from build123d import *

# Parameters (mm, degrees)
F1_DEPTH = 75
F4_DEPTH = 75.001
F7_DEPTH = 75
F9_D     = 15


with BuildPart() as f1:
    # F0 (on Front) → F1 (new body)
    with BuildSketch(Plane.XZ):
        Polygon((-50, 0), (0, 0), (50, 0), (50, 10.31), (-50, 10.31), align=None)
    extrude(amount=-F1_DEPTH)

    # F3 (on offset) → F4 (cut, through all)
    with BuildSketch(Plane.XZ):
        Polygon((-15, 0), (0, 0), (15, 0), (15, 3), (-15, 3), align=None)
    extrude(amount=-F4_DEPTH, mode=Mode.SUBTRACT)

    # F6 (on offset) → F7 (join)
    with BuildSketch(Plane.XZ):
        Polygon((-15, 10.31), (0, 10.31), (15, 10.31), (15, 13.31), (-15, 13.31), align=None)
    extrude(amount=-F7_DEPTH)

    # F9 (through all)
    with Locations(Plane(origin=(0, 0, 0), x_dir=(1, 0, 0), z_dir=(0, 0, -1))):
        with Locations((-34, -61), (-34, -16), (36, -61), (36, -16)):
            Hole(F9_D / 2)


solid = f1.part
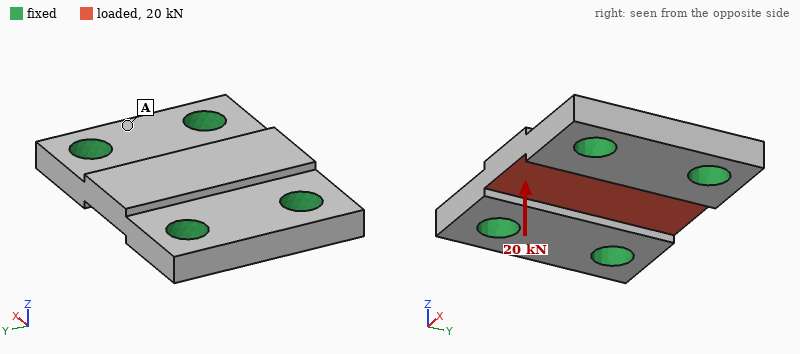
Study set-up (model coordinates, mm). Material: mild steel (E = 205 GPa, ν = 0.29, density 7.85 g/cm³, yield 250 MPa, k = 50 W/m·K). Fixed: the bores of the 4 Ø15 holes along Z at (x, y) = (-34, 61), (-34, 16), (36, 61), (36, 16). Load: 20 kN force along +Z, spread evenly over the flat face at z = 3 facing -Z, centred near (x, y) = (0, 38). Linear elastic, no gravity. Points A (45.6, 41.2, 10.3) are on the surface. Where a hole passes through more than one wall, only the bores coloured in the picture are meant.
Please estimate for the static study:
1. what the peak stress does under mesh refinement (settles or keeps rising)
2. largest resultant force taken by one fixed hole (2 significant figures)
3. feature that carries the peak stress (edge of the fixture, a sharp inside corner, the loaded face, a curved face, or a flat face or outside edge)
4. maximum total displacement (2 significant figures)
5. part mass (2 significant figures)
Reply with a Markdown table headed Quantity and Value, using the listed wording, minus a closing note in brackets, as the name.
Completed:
| Quantity | Value |
|---|---|
| what the peak stress does under mesh refinement | keeps rising |
| largest resultant force taken by one fixed hole | 6.6 kN |
| feature that carries the peak stress | edge of the fixture |
| maximum total displacement | 18 µm |
| part mass | 550 g |
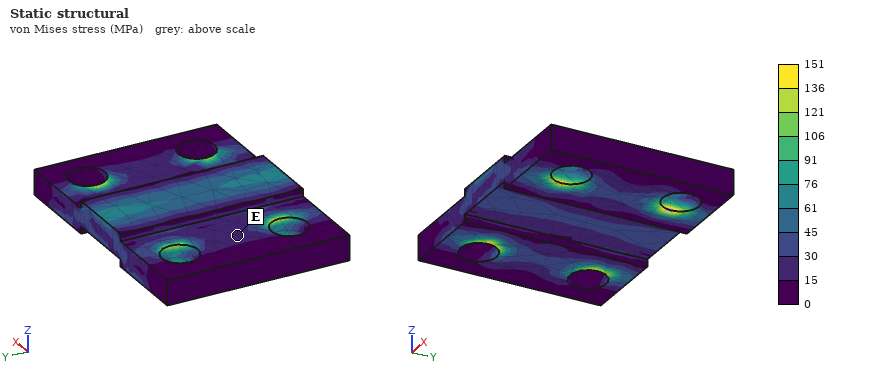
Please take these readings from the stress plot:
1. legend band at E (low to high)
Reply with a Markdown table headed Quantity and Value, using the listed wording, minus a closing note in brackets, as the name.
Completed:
| Quantity | Value |
|---|---|
| legend band at E | 15 to 30 MPa |
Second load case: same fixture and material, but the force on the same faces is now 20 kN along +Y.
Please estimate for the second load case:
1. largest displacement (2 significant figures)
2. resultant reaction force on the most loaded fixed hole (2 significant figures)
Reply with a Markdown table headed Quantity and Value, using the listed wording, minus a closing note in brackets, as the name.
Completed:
| Quantity | Value |
|---|---|
| largest displacement | 7.9 µm |
| resultant reaction force on the most loaded fixed hole | 5.6 kN |
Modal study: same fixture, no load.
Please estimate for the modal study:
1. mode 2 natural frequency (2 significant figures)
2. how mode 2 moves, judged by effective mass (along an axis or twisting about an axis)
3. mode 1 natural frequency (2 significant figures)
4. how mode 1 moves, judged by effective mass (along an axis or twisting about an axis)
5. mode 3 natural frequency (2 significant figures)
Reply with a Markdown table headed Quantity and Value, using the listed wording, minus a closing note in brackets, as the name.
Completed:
| Quantity | Value |
|---|---|
| mode 2 natural frequency | 14 kHz |
| how mode 2 moves, judged by effective mass | twisting about X |
| mode 1 natural frequency | 13 kHz |
| how mode 1 moves, judged by effective mass | along Z |
| mode 3 natural frequency | 18 kHz |
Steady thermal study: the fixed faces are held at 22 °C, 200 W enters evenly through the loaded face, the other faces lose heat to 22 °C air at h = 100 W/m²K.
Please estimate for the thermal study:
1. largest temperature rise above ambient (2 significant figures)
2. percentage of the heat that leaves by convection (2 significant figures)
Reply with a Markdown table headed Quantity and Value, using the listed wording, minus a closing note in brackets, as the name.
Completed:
| Quantity | Value |
|---|---|
| largest temperature rise above ambient | 66 K |
| percentage of the heat that leaves by convection | 15 % |
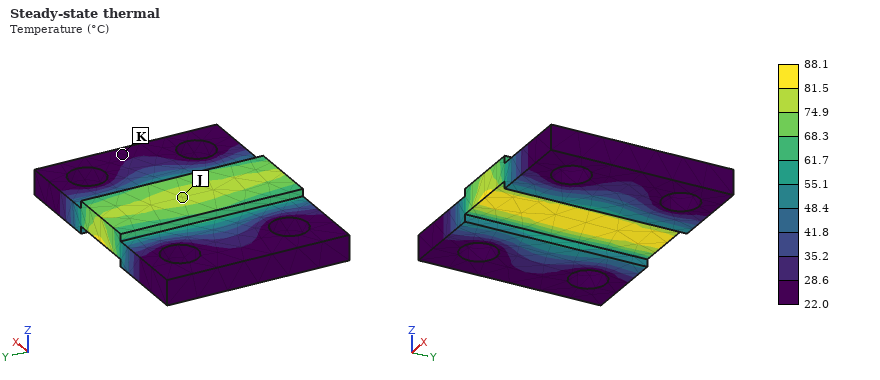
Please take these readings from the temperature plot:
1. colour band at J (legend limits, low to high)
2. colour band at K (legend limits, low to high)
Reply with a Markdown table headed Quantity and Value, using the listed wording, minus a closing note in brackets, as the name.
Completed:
| Quantity | Value |
|---|---|
| colour band at J | 74.9 to 81.5 °C |
| colour band at K | 22.0 to 28.6 °C |
